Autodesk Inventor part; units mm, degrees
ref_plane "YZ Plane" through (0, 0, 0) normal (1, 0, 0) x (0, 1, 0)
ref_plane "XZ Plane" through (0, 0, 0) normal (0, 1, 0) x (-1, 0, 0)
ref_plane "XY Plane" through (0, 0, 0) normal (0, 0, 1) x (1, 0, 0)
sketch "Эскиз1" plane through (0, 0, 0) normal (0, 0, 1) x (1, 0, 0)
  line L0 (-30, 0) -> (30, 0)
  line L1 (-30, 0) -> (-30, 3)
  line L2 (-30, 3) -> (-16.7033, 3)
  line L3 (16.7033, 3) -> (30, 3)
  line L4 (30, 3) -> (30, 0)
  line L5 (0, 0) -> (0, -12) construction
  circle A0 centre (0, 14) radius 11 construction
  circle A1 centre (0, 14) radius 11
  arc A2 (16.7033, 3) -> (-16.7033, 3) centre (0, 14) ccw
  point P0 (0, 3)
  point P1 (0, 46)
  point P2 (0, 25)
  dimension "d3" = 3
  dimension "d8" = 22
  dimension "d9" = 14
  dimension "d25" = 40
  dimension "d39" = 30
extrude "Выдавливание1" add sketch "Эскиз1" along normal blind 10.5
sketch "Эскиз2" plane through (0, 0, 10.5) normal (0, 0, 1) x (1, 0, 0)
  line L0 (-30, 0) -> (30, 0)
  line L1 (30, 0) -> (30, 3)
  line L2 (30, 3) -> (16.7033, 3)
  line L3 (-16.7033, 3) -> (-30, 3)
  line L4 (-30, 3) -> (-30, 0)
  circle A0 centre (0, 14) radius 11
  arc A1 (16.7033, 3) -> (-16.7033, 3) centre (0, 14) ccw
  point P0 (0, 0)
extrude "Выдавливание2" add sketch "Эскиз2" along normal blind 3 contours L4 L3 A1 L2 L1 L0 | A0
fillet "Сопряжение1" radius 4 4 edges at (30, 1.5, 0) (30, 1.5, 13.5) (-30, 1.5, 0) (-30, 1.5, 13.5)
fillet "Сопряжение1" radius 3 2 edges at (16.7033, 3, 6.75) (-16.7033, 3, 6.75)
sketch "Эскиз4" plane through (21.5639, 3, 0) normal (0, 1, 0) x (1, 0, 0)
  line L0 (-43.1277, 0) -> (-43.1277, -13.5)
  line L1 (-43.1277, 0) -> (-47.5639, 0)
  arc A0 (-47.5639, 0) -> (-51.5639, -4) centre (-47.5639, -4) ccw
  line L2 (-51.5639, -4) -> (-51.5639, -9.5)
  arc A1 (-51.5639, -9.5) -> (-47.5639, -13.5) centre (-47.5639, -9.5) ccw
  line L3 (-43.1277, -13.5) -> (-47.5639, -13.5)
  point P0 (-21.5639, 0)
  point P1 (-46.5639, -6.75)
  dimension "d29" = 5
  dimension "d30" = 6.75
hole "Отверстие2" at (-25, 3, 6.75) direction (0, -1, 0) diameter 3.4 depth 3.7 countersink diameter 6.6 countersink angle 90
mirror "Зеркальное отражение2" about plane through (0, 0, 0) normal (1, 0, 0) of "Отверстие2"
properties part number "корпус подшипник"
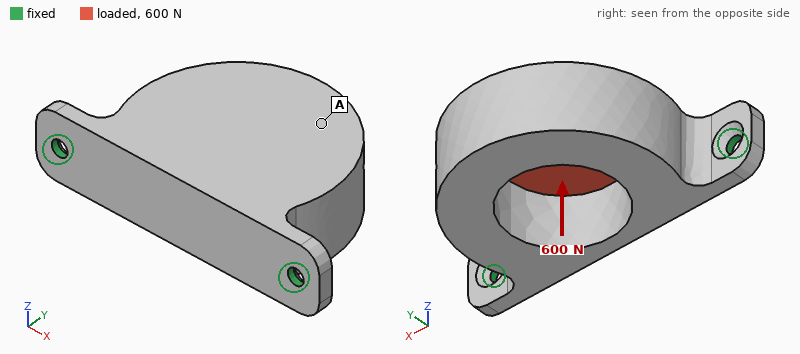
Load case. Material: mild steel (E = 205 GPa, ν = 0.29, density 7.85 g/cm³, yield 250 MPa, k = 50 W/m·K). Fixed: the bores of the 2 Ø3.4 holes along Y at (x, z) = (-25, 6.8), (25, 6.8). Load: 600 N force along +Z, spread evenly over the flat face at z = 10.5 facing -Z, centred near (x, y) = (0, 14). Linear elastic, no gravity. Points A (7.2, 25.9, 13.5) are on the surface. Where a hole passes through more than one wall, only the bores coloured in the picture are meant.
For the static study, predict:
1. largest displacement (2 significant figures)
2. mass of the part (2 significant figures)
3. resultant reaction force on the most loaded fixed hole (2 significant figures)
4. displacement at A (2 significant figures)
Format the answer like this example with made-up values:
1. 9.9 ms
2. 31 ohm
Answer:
1. 0.12 mm
2. 99 g
3. 300 N
4. 0.092 mm
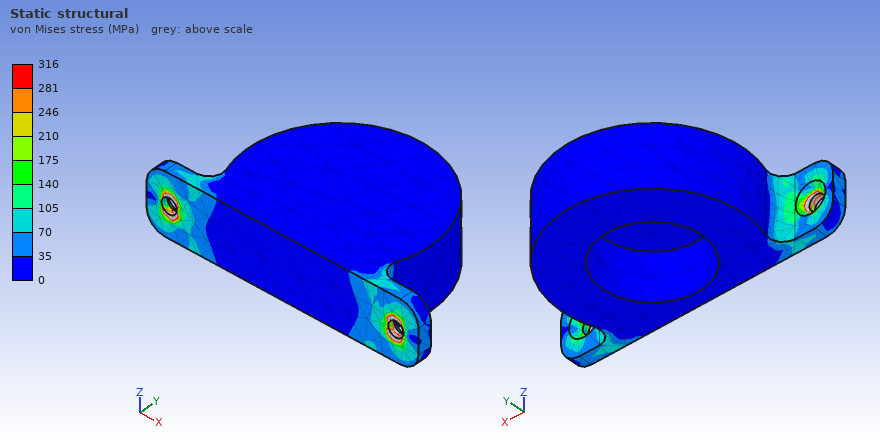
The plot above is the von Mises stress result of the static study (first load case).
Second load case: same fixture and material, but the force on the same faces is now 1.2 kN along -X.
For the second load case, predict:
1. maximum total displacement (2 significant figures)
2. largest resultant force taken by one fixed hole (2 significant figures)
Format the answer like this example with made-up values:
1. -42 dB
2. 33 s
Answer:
1. 4.8 µm
2. 690 N
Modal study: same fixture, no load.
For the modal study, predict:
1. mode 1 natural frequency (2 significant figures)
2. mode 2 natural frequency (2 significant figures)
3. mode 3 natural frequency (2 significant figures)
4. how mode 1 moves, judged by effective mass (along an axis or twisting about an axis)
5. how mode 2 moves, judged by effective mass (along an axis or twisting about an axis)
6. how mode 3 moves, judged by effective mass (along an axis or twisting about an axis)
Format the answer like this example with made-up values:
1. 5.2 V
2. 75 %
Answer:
1. 1300 Hz
2. 7500 Hz
3. 7800 Hz
4. along Z
5. along Y
6. along X
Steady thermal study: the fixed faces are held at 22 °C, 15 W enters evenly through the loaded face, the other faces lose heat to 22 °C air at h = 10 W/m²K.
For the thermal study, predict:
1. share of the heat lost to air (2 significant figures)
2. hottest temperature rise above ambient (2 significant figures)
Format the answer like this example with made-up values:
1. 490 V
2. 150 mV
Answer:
1. 12 %
2. 51 K
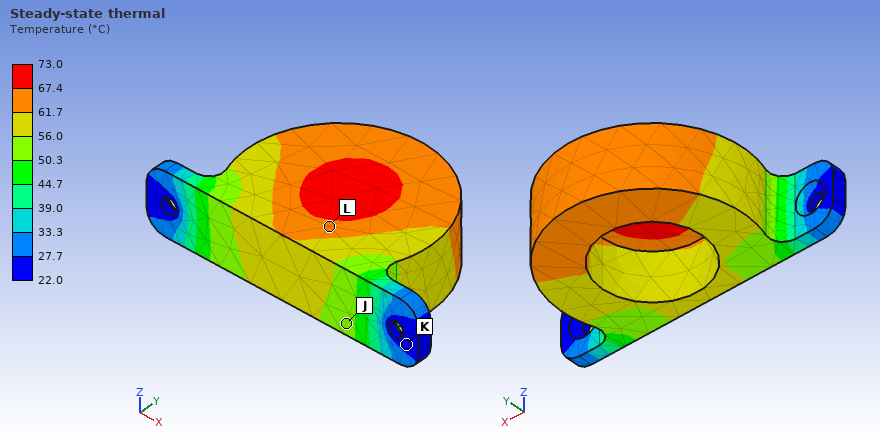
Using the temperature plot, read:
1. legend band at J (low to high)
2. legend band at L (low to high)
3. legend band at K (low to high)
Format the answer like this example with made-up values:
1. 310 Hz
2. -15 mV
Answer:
1. 50.3 to 56.0 °C
2. 61.7 to 67.4 °C
3. 22.0 to 27.7 °C
